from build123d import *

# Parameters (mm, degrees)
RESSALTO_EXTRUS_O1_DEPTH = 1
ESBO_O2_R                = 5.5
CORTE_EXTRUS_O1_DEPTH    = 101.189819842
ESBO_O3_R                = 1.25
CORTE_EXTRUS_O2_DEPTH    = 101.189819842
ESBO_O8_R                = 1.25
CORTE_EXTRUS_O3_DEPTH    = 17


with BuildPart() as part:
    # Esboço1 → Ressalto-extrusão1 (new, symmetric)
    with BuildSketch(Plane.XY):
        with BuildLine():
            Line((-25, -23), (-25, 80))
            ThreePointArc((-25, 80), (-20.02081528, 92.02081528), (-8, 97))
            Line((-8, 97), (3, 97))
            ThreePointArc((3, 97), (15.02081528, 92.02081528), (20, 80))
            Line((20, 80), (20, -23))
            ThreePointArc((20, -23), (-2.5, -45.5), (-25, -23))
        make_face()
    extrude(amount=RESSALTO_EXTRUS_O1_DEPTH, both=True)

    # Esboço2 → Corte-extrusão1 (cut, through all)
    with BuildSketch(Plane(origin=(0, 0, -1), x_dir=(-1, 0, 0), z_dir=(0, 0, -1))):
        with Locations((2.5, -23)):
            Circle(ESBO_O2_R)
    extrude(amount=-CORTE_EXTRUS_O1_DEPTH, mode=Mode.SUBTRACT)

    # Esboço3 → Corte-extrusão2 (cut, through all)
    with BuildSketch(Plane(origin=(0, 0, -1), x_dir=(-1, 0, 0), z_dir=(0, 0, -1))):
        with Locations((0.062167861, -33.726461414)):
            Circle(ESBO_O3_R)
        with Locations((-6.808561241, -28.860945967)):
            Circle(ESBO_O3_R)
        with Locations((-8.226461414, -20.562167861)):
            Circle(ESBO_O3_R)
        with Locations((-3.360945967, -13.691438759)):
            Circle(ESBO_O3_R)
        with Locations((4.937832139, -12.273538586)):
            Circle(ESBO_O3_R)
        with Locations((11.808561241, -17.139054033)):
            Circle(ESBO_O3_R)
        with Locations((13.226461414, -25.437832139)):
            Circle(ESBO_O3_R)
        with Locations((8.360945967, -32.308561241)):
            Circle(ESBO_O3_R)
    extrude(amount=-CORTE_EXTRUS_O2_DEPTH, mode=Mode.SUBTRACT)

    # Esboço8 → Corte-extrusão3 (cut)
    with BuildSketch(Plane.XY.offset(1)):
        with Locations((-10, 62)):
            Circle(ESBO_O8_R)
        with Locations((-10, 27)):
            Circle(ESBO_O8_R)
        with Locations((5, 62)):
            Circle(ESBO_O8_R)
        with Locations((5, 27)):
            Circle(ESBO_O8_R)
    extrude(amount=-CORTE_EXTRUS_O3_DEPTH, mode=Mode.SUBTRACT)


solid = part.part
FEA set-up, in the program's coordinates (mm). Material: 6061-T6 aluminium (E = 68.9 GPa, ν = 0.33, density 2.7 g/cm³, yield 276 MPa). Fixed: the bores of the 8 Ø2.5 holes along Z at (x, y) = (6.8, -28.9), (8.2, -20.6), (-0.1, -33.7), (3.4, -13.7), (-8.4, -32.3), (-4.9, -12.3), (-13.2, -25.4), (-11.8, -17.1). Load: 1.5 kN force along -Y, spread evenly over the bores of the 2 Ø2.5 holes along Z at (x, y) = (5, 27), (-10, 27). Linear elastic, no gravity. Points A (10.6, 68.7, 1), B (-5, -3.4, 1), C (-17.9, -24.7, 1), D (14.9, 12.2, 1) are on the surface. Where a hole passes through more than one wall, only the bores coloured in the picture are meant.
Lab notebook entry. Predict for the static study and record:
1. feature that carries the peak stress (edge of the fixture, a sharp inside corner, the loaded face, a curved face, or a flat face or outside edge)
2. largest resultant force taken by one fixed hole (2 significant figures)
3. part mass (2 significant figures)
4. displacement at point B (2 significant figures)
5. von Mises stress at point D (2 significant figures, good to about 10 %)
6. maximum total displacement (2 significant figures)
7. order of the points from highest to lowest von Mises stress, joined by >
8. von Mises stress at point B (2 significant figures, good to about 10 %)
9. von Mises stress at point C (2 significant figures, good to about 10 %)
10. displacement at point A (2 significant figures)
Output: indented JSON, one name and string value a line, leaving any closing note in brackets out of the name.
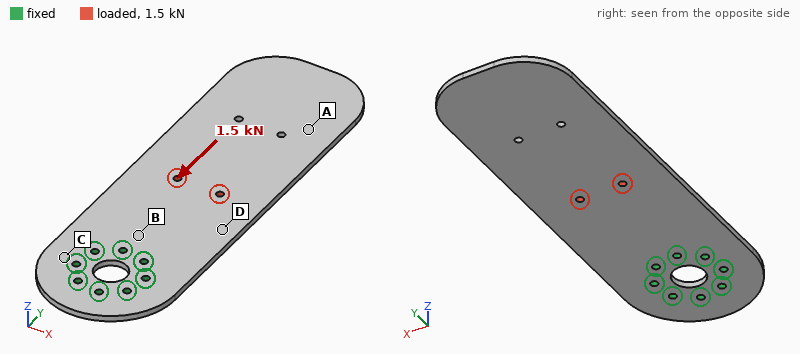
{
  "feature that carries the peak stress": "the loaded face",
  "largest resultant force taken by one fixed hole": "380 N",
  "part mass": "32 g",
  "displacement at point B": "3.1 µm",
  "von Mises stress at point D": "14 MPa",
  "maximum total displacement": "14 µm",
  "order of the points from highest to lowest von Mises stress, joined by >": "B > D > C > A",
  "von Mises stress at point B": "23 MPa",
  "von Mises stress at point C": "7.2 MPa",
  "displacement at point A": "11 µm"
}
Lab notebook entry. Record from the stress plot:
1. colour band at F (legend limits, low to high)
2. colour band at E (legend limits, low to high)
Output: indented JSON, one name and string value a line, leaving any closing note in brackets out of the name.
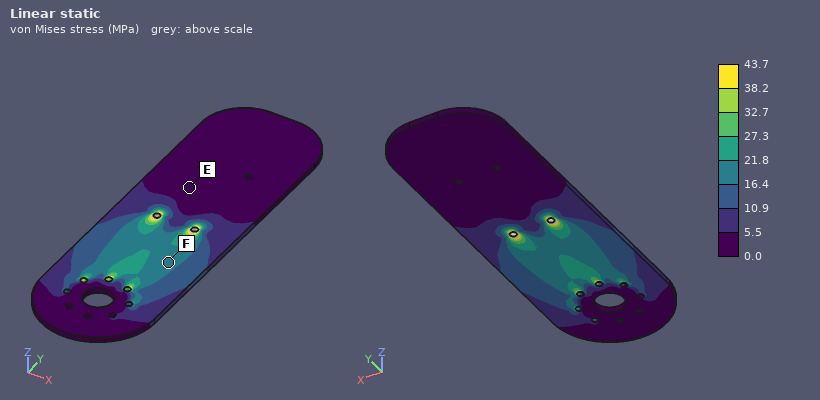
{
  "colour band at F": "16.4 to 21.8 MPa",
  "colour band at E": "0.0 to 5.5 MPa"
}
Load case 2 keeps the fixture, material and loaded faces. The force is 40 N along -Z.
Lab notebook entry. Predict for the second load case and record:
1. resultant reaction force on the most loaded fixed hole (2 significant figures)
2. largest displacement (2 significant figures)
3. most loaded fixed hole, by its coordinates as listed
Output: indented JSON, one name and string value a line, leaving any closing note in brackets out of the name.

{
  "resultant reaction force on the most loaded fixed hole": "75 N",
  "largest displacement": "1.5 mm",
  "most loaded fixed hole, by its coordinates as listed": "(-4.9, -12.3)"
}
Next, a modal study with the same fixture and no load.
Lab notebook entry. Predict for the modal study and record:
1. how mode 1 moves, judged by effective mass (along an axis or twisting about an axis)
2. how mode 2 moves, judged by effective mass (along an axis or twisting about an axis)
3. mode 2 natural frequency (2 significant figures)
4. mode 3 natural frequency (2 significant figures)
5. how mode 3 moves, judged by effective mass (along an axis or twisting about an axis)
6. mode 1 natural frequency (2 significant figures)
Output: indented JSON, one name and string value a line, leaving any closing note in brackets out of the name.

{
  "how mode 1 moves, judged by effective mass": "along Z",
  "how mode 2 moves, judged by effective mass": "twisting about Y",
  "mode 2 natural frequency": "690 Hz",
  "mode 3 natural frequency": "870 Hz",
  "how mode 3 moves, judged by effective mass": "along Z",
  "mode 1 natural frequency": "140 Hz"
}
